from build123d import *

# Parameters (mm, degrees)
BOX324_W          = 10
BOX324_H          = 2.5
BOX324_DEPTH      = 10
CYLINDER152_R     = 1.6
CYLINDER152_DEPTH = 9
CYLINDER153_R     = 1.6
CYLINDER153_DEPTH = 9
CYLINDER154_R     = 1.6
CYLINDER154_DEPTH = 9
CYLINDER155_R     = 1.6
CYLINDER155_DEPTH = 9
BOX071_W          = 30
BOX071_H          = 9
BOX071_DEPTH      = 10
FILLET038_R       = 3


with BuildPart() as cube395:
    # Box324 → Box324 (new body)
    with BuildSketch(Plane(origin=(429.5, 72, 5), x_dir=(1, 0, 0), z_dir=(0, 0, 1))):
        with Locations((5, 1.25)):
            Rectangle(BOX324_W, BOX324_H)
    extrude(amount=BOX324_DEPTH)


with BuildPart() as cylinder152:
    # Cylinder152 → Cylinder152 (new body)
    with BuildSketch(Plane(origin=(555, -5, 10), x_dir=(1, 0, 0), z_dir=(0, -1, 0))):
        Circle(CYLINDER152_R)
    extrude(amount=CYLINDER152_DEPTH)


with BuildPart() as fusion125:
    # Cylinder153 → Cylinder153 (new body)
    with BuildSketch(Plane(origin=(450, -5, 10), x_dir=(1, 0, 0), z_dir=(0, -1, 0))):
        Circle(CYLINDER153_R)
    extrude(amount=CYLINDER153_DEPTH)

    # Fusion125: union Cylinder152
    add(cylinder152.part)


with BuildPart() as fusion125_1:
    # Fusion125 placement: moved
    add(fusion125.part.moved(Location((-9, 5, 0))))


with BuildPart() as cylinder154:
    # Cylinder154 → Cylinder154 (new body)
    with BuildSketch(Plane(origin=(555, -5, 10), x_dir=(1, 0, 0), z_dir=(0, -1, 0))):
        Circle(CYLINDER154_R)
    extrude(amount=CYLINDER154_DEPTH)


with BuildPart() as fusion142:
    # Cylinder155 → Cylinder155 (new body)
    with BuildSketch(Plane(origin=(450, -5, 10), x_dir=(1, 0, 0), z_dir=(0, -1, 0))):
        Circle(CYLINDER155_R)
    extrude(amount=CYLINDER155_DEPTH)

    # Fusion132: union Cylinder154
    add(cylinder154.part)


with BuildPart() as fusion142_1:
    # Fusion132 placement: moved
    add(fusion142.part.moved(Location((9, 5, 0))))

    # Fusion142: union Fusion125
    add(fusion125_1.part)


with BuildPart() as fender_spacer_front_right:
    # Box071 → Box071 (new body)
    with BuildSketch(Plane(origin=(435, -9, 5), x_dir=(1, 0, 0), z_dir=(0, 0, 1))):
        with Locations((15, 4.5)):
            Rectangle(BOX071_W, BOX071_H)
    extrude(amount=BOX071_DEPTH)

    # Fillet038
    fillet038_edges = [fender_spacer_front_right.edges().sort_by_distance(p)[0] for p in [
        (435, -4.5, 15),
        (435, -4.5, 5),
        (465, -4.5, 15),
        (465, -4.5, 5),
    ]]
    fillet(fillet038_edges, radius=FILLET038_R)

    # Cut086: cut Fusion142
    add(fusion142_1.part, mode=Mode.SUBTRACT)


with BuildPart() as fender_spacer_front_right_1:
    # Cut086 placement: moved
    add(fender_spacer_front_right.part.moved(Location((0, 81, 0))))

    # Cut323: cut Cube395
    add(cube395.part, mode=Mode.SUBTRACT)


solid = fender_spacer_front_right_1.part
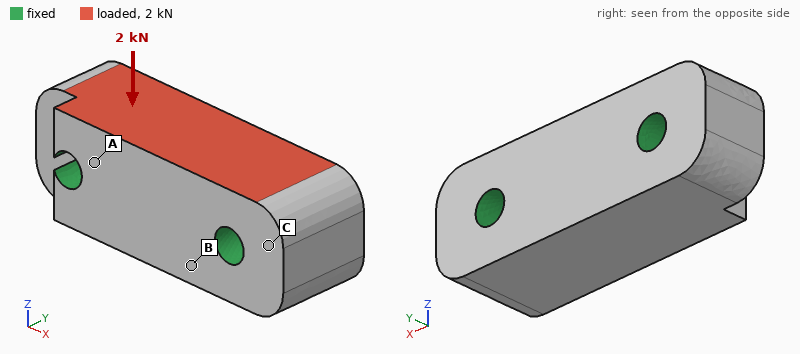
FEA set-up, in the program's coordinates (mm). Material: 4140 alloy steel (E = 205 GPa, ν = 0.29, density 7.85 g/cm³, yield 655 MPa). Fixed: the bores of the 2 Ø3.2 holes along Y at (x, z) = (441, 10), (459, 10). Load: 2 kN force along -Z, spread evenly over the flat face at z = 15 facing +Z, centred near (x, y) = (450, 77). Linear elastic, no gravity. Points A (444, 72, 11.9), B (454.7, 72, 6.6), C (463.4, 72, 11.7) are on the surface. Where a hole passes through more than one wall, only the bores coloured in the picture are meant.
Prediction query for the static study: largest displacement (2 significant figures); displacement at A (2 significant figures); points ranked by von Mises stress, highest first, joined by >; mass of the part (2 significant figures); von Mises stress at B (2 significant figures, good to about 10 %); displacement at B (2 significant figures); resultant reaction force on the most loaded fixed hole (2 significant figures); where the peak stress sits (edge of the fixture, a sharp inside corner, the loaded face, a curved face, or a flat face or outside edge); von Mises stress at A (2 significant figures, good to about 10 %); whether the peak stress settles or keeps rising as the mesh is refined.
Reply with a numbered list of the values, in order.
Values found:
1. 0.89 µm
2. 0.37 µm
3. A > B > C
4. 19 g
5. 8.8 MPa
6. 0.43 µm
7. 1.0 kN
8. edge of the fixture
9. 15 MPa
10. keeps rising
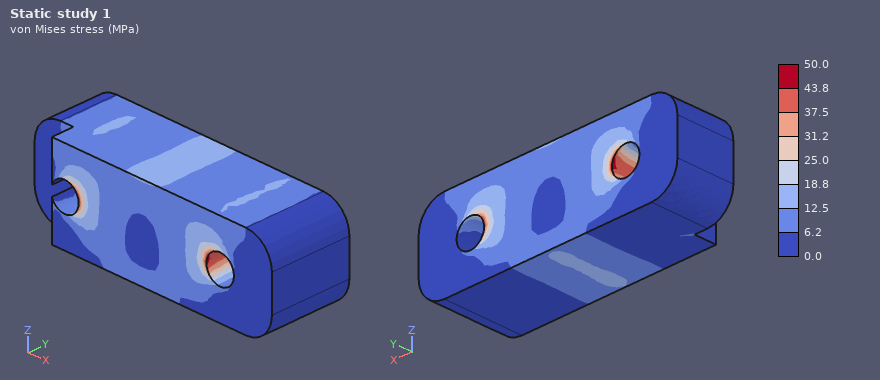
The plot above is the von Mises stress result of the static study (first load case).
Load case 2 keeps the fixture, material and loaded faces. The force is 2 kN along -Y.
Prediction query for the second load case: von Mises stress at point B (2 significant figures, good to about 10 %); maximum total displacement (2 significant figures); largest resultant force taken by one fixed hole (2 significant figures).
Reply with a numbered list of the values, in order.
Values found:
1. 14 MPa
2. 2.5 µm
3. 1.0 kN
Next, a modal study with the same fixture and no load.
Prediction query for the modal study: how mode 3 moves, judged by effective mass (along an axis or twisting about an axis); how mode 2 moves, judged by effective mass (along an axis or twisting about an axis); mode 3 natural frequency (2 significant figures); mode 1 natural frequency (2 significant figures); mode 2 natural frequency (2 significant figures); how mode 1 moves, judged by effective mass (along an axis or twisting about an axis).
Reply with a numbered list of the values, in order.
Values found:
1. twisting about X
2. along Y
3. 81 kHz
4. 67 kHz
5. 74 kHz
6. along Z
